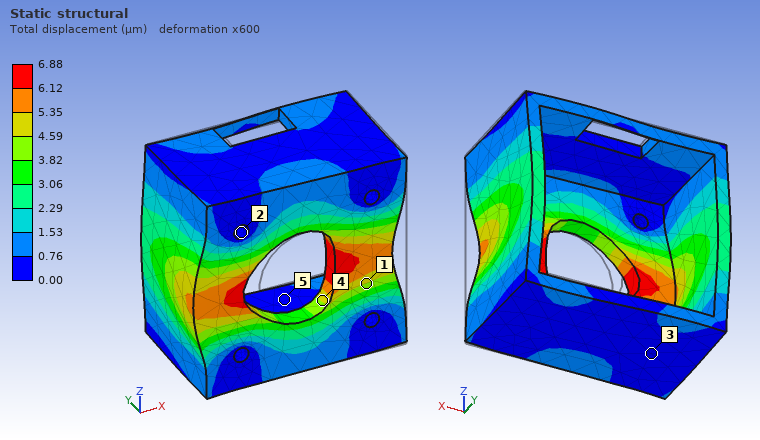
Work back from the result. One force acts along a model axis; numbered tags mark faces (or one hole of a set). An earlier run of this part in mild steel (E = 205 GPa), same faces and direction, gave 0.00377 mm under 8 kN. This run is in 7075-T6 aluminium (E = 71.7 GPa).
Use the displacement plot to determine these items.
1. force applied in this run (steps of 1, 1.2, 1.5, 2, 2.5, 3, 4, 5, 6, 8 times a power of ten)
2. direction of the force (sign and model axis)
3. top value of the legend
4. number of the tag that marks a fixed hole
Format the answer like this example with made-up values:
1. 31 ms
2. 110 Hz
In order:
1. 5 kN
2. -X
3. 6.88 µm
4. 2
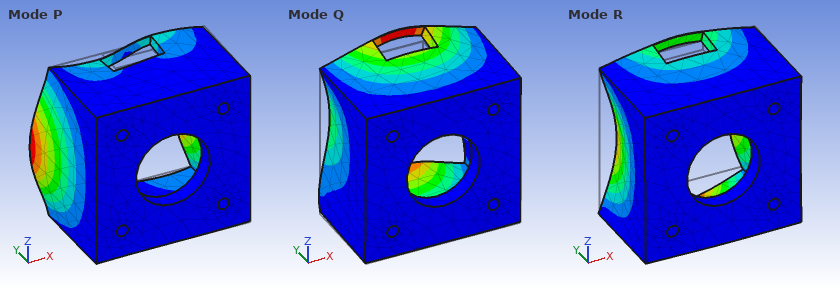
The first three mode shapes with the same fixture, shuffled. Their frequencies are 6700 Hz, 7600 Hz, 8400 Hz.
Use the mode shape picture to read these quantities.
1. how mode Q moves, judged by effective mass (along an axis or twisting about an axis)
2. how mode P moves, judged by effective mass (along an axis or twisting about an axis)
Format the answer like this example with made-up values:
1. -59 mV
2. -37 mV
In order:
1. along Z
2. along X
